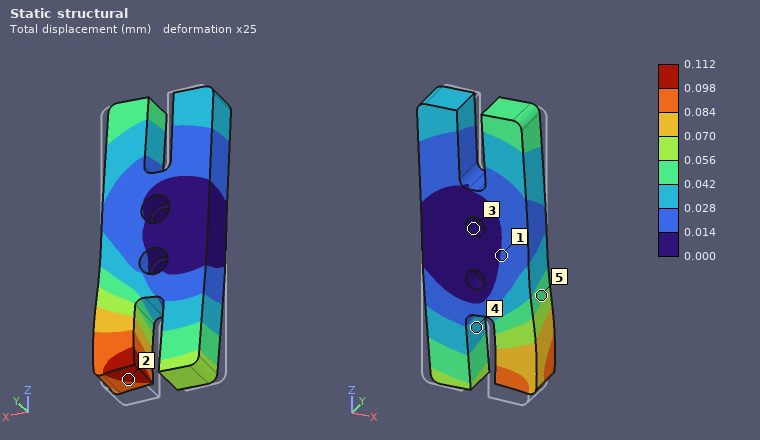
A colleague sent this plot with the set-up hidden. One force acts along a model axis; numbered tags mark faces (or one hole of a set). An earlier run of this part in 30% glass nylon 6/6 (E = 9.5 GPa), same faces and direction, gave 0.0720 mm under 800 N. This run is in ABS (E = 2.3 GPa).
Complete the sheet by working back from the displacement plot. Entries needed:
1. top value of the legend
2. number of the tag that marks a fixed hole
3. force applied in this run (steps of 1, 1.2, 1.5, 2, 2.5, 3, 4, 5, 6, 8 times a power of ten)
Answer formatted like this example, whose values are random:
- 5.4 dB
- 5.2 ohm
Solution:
- 0.112 mm
- 3
- 300 N
